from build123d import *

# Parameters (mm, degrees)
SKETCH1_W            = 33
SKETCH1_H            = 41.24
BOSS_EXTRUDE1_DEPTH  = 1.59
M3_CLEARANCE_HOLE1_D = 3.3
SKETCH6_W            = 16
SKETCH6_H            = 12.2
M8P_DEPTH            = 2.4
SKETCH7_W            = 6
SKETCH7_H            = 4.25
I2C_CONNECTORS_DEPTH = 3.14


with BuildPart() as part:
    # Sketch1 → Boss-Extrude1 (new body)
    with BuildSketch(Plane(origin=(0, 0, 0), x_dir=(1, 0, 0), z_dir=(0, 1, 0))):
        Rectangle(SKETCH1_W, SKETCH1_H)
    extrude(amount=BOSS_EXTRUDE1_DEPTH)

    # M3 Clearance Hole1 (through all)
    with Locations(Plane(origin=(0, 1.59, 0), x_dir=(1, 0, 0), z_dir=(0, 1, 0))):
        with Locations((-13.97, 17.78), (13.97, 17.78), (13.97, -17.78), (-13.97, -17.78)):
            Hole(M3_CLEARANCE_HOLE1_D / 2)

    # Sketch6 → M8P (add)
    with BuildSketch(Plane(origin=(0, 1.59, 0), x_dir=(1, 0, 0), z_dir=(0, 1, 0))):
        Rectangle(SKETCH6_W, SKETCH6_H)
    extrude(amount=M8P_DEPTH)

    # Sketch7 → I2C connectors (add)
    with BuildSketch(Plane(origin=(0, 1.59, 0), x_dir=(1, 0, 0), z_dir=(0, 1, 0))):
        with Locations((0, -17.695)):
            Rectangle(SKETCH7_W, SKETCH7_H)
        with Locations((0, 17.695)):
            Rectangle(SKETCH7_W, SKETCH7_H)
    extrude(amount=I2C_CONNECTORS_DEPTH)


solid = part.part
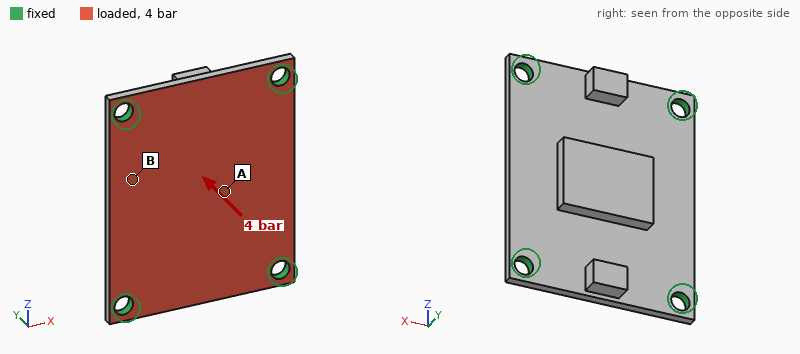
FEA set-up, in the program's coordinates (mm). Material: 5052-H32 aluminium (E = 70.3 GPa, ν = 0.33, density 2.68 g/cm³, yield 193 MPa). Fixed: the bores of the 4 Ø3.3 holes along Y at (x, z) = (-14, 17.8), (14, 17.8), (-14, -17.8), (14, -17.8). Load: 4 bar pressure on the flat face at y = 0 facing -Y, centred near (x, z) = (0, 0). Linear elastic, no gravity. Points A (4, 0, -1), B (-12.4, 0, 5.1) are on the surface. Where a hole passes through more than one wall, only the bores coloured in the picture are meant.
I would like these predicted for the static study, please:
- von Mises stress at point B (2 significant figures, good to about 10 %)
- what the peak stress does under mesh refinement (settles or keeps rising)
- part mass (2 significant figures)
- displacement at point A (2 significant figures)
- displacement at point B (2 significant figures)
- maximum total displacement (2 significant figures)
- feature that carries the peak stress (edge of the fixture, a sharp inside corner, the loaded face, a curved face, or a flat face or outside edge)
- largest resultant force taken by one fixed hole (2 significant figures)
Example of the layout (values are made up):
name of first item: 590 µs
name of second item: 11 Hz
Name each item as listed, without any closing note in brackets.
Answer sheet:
von Mises stress at point B: 43 MPa
what the peak stress does under mesh refinement: keeps rising
part mass: 7.3 g
displacement at point A: 61 µm
displacement at point B: 54 µm
maximum total displacement: 62 µm
feature that carries the peak stress: edge of the fixture
largest resultant force taken by one fixed hole: 140 N
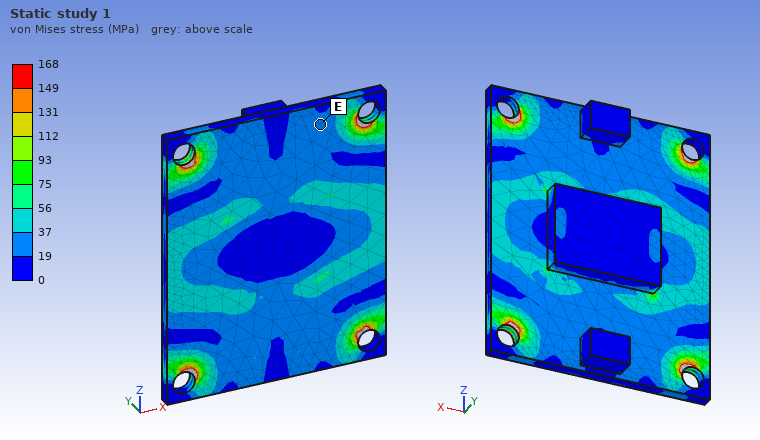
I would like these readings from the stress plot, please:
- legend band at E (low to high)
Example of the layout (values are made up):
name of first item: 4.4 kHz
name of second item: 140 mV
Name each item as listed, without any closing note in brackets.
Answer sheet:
legend band at E: 19 to 37 MPa
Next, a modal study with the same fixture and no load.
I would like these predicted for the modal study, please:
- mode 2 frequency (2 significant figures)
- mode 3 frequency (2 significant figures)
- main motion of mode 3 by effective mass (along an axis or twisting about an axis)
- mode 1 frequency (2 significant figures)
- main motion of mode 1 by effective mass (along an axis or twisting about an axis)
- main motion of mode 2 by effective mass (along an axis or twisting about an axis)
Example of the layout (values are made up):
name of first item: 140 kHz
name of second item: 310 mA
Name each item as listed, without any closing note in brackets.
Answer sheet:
mode 2 frequency: 8900 Hz
mode 3 frequency: 11 kHz
main motion of mode 3 by effective mass: twisting about X
mode 1 frequency: 5600 Hz
main motion of mode 1 by effective mass: along Y
main motion of mode 2 by effective mass: twisting about Z
